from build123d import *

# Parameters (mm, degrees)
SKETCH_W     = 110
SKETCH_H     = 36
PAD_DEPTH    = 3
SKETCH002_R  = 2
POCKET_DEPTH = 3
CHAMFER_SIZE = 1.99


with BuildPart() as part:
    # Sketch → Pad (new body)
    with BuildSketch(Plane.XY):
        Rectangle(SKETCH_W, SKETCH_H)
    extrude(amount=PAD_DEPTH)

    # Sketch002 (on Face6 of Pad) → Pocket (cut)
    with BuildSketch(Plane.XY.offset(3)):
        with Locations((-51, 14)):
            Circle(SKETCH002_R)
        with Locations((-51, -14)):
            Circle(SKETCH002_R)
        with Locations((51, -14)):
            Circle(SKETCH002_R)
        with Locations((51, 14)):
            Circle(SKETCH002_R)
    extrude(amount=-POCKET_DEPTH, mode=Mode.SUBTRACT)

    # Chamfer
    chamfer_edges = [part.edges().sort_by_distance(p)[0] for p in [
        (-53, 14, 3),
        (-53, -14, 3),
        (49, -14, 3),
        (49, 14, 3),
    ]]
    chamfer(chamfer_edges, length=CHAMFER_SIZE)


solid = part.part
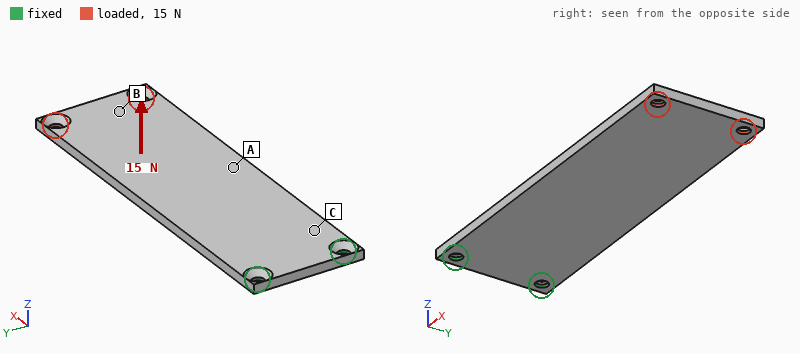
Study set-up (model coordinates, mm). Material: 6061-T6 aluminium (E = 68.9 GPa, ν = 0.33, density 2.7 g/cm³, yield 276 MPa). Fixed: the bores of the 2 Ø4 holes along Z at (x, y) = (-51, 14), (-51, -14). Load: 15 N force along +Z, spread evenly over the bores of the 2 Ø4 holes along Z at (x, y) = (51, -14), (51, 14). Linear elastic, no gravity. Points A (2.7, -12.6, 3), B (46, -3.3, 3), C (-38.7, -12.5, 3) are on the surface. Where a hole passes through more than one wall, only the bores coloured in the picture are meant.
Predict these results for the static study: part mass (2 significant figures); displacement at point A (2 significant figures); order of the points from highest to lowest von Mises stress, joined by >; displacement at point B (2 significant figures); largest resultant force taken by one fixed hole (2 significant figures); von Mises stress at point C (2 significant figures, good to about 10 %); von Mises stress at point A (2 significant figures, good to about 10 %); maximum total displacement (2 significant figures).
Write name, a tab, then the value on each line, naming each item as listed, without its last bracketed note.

part mass	31 g
displacement at point A	0.46 mm
order of the points from highest to lowest von Mises stress, joined by >	C > A > B
displacement at point B	1.1 mm
largest resultant force taken by one fixed hole	9.1 N
von Mises stress at point C	24 MPa
von Mises stress at point A	13 MPa
maximum total displacement	1.3 mm
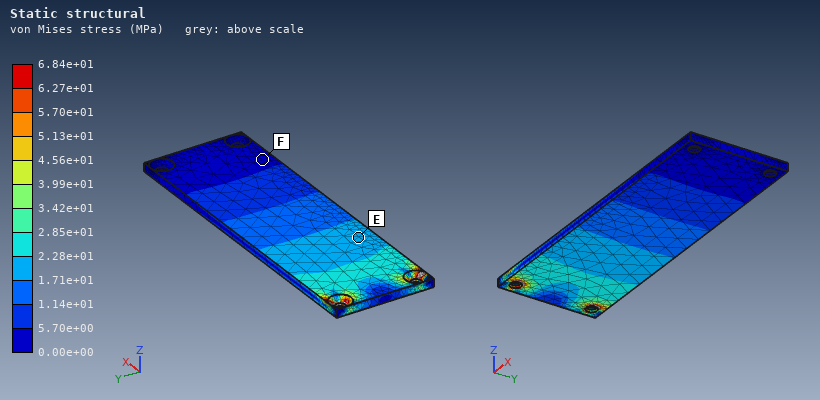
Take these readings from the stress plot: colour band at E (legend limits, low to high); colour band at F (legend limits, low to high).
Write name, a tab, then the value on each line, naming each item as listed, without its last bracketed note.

colour band at E	1.71e+01 to 2.28e+01 MPa
colour band at F	0.00e+00 to 5.70e+00 MPa
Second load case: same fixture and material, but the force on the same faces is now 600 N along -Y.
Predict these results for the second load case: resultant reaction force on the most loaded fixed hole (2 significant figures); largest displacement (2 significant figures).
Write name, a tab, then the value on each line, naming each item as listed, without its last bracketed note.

resultant reaction force on the most loaded fixed hole	2.1 kN
largest displacement	0.43 mm
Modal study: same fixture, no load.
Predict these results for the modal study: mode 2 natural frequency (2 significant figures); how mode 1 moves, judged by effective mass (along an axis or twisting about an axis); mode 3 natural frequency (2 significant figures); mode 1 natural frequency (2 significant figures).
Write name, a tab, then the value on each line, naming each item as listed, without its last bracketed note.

mode 2 natural frequency	1300 Hz
how mode 1 moves, judged by effective mass	along Z
mode 3 natural frequency	1300 Hz
mode 1 natural frequency	190 Hz
